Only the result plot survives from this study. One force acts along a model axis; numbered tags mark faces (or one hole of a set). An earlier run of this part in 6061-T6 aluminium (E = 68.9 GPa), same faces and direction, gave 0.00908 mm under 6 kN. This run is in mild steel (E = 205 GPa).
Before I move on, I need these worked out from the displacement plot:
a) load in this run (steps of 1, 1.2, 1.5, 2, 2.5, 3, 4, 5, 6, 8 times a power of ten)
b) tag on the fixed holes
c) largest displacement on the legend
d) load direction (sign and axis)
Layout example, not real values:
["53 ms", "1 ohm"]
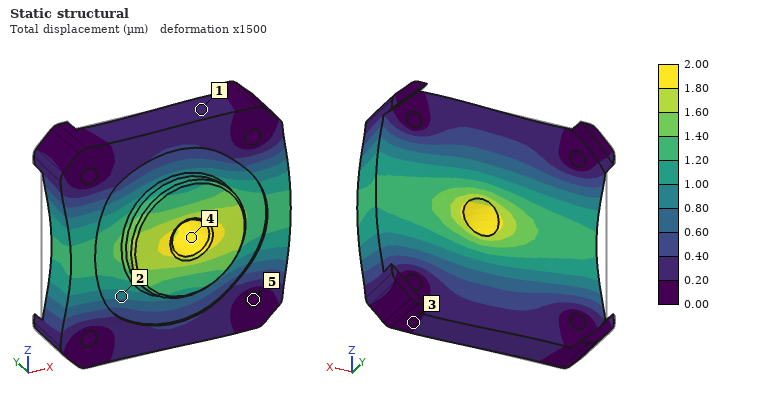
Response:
["4 kN", "5", "2.00 µm", "+X"]
